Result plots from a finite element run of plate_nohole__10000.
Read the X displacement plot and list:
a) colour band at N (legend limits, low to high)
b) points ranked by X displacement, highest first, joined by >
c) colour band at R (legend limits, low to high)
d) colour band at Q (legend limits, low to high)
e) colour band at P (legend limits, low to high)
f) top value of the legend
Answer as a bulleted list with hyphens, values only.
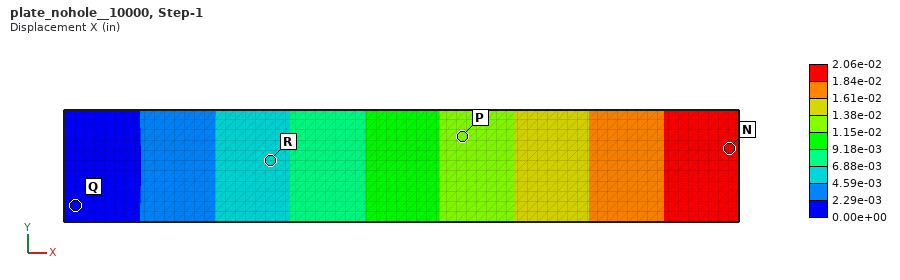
- 1.84e-02 to 2.06e-02 in
- N > P > R > Q
- 4.59e-03 to 6.88e-03 in
- 0.00e+00 to 2.29e-03 in
- 1.15e-02 to 1.38e-02 in
- 2.06e-02 in
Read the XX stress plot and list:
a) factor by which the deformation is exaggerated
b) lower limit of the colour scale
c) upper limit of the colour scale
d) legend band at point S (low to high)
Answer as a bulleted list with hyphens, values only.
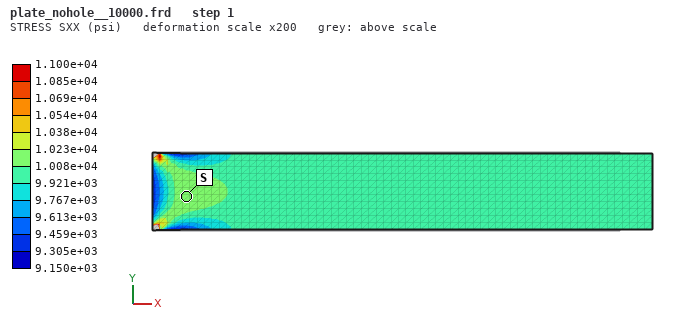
- 200
- 9.150e+03 psi
- 1.100e+04 psi
- 1.008e+04 to 1.023e+04 psi
